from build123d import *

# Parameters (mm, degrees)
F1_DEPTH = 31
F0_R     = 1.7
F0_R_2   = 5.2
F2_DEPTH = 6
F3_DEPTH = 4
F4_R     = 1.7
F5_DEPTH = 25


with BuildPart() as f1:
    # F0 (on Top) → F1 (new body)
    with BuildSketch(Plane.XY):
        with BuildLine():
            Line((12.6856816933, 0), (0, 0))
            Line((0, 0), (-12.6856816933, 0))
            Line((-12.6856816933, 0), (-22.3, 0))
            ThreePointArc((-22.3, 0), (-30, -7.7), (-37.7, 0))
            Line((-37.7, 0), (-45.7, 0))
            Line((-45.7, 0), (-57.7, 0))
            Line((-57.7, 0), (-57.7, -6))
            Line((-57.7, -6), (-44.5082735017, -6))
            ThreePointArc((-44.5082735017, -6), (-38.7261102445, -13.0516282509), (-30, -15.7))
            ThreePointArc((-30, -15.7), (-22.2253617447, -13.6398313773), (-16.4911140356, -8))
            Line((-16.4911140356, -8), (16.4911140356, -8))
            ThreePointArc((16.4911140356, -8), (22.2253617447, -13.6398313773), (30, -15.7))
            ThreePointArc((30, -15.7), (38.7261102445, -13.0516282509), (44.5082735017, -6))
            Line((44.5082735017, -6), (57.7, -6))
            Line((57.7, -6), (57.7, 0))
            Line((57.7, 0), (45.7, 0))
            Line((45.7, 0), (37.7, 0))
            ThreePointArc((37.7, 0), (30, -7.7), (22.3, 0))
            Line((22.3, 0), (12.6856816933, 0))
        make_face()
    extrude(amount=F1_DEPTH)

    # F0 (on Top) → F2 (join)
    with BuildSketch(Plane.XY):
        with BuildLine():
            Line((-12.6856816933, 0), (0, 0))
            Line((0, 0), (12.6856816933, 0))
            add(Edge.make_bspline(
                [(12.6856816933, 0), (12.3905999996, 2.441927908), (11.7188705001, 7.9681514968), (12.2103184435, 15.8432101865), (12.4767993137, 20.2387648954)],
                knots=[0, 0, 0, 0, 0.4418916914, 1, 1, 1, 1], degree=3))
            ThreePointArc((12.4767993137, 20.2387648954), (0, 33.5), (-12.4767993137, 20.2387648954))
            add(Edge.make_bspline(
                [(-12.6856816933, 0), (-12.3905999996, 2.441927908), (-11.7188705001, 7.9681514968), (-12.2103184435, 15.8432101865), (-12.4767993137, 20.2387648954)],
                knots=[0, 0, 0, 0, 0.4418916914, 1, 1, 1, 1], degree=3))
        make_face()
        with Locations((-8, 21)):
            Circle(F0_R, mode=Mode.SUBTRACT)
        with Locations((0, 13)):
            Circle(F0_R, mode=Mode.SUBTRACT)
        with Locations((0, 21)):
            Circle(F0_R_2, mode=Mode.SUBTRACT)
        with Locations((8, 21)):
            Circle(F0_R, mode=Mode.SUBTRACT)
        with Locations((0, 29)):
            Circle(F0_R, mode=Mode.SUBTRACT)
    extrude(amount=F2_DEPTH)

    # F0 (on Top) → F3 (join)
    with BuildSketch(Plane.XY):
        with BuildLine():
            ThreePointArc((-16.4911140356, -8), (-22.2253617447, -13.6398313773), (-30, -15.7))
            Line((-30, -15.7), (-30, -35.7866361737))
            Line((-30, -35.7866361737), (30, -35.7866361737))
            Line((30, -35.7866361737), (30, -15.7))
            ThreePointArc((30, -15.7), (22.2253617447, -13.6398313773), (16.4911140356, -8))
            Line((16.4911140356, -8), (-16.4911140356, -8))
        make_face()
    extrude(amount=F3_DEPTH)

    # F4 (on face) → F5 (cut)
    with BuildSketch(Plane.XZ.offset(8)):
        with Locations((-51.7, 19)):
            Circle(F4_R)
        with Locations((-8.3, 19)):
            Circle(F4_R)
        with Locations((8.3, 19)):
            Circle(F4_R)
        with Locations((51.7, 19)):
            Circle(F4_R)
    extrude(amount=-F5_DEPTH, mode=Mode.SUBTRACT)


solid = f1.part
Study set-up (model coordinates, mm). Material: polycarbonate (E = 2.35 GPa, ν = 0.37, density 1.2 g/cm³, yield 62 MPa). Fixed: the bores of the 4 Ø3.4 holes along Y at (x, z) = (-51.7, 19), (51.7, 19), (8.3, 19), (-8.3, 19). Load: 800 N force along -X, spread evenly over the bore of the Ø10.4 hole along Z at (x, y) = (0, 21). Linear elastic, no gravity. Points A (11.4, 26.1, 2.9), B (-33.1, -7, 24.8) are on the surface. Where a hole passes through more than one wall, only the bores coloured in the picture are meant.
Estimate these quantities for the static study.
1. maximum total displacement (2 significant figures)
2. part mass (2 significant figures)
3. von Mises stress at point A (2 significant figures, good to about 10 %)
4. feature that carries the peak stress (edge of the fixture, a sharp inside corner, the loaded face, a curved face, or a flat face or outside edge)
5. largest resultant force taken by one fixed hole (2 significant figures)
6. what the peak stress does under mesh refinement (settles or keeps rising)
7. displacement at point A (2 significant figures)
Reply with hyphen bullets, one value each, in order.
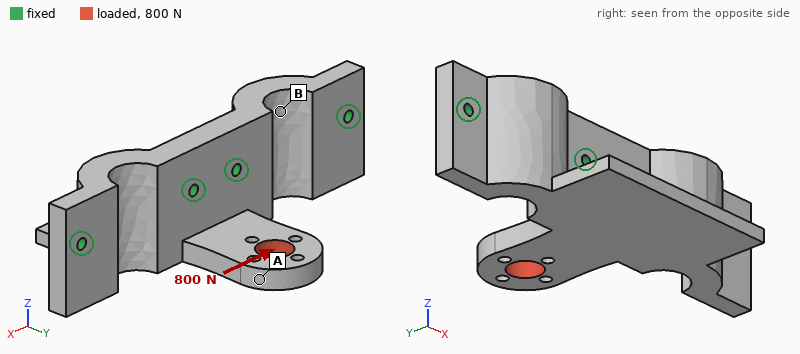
- 1.4 mm
- 48 g
- 11 MPa
- edge of the fixture
- 790 N
- keeps rising
- 1.2 mm
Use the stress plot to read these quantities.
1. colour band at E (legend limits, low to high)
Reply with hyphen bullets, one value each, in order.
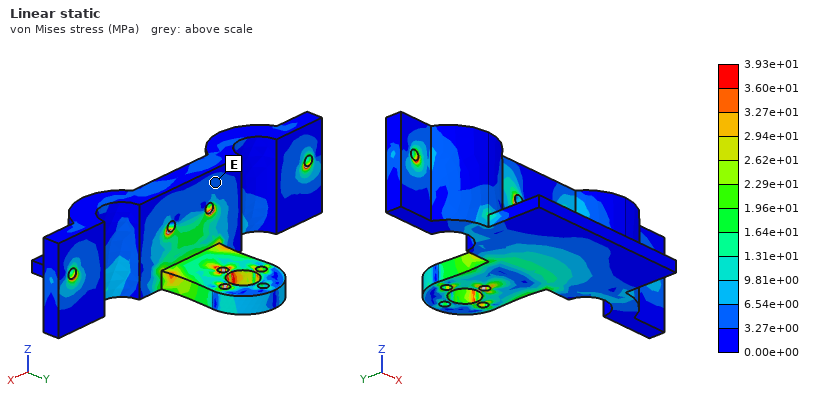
- 3.27e+00 to 6.54e+00 MPa
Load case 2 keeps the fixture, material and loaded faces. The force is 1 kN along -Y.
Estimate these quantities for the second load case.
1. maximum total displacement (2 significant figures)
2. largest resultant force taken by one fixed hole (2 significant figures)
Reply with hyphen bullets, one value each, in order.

- 1.2 mm
- 440 N
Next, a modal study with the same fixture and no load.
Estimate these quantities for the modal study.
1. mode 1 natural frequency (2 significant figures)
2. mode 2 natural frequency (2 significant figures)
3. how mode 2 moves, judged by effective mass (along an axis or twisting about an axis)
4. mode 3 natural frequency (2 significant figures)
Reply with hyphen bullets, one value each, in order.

- 970 Hz
- 1300 Hz
- along Z
- 1600 Hz
